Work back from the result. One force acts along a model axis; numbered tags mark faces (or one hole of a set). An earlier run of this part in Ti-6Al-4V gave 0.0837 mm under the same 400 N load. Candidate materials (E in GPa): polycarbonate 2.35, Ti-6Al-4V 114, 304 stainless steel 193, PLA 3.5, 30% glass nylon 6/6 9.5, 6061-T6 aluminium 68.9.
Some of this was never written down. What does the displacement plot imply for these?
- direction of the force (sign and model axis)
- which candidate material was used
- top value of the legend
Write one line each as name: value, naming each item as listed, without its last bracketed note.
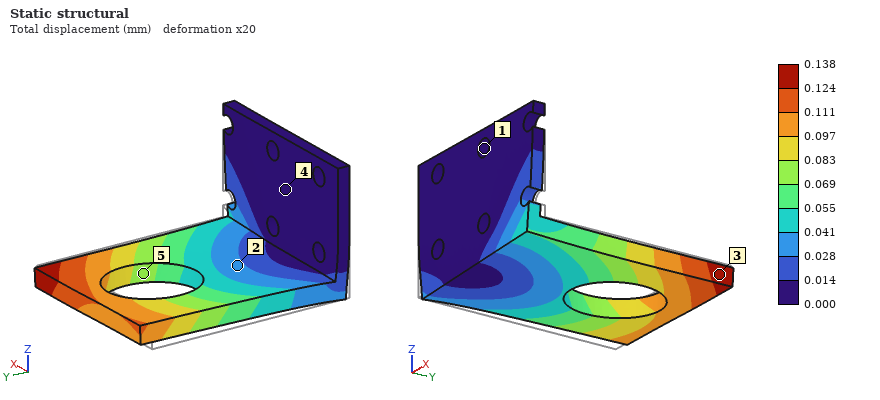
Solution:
direction of the force: +X
which candidate material was used: 6061-T6 aluminium
top value of the legend: 0.138 mm
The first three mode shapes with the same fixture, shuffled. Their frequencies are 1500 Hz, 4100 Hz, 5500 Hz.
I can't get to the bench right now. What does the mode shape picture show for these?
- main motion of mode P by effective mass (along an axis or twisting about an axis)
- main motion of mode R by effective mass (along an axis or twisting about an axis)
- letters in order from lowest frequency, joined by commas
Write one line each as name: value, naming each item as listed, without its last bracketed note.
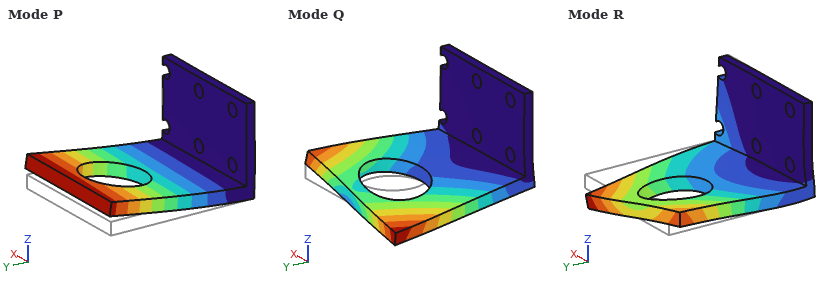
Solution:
main motion of mode P by effective mass: along Z
main motion of mode R by effective mass: along X
letters in order from lowest frequency, joined by commas: P, Q, R
